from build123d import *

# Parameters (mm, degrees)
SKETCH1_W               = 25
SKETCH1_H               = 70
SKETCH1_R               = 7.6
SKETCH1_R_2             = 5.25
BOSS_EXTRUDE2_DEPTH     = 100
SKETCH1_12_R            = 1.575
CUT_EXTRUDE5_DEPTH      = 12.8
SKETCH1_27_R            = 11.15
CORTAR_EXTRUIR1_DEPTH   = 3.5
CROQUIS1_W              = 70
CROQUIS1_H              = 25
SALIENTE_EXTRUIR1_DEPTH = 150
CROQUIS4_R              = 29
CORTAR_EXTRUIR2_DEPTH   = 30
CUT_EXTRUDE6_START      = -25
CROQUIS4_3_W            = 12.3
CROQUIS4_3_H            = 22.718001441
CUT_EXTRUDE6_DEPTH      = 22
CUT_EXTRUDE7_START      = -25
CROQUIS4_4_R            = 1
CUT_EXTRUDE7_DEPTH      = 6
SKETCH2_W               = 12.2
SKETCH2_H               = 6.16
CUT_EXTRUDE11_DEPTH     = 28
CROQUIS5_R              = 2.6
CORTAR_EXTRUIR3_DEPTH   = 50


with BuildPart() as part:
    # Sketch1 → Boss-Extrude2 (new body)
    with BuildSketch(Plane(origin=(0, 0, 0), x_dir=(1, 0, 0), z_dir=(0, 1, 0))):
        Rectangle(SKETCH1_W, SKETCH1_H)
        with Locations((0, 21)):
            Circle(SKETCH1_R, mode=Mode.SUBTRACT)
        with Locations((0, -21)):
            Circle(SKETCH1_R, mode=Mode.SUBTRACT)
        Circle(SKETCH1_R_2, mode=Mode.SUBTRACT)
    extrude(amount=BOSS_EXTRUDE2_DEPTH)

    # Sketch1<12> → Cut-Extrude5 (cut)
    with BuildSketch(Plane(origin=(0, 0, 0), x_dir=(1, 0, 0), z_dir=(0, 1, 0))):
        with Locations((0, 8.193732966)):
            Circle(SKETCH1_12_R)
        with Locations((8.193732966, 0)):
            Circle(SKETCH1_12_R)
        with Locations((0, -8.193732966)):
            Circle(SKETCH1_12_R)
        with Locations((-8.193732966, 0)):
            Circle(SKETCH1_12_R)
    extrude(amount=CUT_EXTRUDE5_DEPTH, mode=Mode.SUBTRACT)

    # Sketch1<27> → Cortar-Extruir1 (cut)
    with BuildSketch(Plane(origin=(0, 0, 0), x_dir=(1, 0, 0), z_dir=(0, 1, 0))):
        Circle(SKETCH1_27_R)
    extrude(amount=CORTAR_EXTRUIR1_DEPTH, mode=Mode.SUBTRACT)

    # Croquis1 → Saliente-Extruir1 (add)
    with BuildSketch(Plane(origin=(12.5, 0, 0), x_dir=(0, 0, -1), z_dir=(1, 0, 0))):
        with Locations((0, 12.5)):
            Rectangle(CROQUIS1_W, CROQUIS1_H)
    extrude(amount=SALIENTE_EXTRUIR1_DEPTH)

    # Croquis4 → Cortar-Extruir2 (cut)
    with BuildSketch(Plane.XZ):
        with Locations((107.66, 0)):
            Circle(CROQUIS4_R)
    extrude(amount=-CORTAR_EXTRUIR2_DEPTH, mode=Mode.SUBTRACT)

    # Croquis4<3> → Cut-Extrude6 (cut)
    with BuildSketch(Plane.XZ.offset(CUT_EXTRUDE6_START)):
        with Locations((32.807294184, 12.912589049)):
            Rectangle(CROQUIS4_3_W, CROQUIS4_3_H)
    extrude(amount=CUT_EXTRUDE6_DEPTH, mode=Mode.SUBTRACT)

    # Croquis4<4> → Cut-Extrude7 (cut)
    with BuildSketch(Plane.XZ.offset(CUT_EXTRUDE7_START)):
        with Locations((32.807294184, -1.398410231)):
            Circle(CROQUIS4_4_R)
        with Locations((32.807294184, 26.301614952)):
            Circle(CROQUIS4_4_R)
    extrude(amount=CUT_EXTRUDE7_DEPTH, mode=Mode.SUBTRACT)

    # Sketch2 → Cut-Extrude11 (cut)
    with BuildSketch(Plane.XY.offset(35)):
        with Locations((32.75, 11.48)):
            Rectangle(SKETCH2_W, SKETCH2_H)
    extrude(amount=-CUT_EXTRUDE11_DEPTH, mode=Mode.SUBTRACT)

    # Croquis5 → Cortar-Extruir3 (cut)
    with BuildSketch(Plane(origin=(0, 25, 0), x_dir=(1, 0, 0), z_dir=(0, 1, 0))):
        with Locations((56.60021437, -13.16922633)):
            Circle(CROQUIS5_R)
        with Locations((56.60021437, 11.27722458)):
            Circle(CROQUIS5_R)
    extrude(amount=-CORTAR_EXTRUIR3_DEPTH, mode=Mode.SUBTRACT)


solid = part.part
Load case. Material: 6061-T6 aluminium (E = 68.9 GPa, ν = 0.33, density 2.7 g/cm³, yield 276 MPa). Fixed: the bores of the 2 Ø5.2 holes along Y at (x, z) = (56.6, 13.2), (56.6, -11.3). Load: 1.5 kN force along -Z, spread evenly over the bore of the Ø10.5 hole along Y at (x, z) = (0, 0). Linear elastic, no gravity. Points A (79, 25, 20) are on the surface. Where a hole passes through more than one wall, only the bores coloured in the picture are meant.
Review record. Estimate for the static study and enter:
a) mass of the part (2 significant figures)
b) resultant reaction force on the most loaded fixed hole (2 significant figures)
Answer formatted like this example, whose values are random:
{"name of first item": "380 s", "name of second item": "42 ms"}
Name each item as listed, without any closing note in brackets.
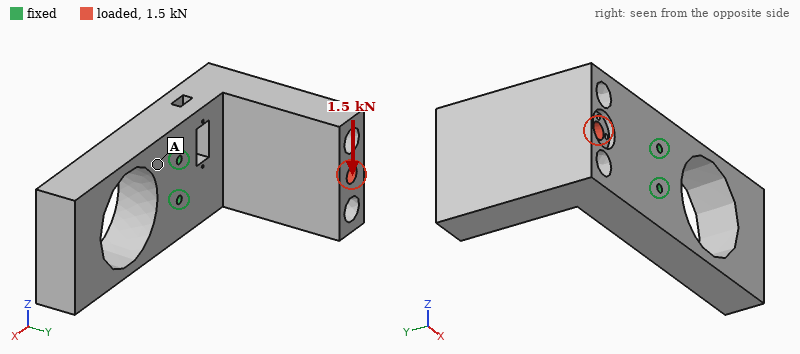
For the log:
{"mass of the part": "860 g", "resultant reaction force on the most loaded fixed hole": "3.3 kN"}
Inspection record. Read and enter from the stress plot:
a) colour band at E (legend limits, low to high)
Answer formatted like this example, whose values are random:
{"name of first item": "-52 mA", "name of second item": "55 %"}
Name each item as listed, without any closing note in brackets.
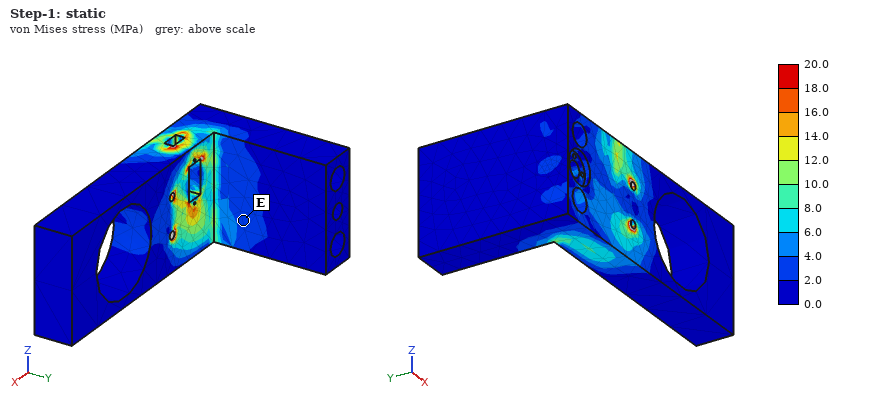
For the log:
{"colour band at E": "2.0 to 4.0 MPa"}
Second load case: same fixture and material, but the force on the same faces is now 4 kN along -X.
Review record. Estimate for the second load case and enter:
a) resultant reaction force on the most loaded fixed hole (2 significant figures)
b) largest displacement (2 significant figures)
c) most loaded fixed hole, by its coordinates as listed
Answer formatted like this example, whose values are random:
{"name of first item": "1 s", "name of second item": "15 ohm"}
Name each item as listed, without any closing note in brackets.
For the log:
{"resultant reaction force on the most loaded fixed hole": "2.3 kN", "largest displacement": "0.24 mm", "most loaded fixed hole, by its coordinates as listed": "(56.6, -11.3)"}
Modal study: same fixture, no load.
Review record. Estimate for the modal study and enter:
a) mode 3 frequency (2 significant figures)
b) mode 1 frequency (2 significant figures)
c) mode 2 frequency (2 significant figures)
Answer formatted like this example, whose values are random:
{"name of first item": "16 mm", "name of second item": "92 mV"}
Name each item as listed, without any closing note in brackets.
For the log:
{"mode 3 frequency": "1500 Hz", "mode 1 frequency": "1100 Hz", "mode 2 frequency": "1300 Hz"}
